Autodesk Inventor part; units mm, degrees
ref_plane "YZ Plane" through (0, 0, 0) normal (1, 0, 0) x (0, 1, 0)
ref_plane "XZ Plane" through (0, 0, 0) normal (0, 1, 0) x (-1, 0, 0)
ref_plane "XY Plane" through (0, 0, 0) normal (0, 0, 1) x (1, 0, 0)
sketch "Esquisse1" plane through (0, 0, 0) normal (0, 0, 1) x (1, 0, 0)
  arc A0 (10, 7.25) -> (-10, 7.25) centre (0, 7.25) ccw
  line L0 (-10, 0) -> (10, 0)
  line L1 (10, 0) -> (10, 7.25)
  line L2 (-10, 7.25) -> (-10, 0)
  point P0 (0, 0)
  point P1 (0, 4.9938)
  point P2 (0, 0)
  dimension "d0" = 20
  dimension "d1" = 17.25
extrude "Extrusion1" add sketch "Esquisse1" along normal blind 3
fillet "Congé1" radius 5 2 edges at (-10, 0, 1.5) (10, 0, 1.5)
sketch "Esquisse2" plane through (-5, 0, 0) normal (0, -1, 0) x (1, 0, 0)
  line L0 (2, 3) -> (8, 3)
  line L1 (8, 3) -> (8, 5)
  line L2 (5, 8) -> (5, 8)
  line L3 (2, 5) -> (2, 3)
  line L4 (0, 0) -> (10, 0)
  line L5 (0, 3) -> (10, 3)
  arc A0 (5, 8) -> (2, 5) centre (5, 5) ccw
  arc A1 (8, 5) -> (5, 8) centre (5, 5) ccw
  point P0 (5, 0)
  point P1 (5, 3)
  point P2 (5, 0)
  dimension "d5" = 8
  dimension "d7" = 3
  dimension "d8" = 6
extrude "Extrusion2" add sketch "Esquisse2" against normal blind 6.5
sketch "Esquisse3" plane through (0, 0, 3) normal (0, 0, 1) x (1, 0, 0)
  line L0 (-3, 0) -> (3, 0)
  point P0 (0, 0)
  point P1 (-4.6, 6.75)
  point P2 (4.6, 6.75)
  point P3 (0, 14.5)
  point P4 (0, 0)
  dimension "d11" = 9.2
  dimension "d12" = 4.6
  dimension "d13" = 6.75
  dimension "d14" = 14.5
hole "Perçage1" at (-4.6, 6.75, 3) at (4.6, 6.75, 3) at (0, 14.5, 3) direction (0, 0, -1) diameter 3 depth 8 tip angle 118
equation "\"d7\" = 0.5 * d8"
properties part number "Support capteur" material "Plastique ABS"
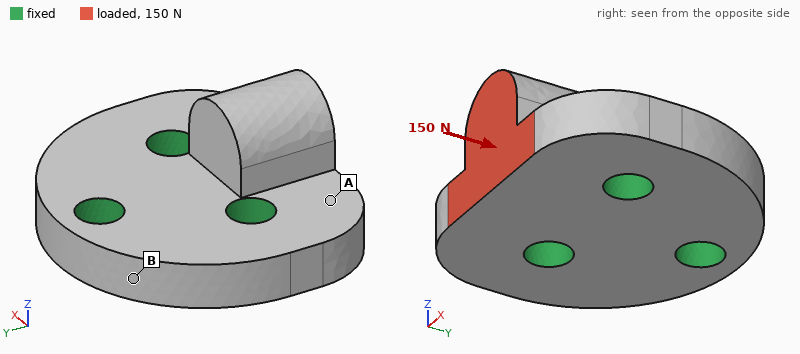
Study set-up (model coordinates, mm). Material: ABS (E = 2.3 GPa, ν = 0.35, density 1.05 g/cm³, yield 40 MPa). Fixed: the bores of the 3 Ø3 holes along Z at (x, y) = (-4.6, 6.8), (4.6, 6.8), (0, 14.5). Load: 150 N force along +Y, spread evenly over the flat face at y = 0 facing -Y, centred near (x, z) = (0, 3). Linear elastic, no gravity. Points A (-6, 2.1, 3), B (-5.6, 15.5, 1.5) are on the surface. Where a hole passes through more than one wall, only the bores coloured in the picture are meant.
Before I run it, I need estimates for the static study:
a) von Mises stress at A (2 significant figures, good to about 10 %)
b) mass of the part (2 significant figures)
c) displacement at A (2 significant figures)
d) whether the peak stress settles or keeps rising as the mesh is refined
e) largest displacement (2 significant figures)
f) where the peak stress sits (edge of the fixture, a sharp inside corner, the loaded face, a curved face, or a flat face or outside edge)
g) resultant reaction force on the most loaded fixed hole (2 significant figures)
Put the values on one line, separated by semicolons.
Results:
3.4 MPa; 1.0 g; 16 µm; keeps rising; 74 µm; edge of the fixture; 72 N
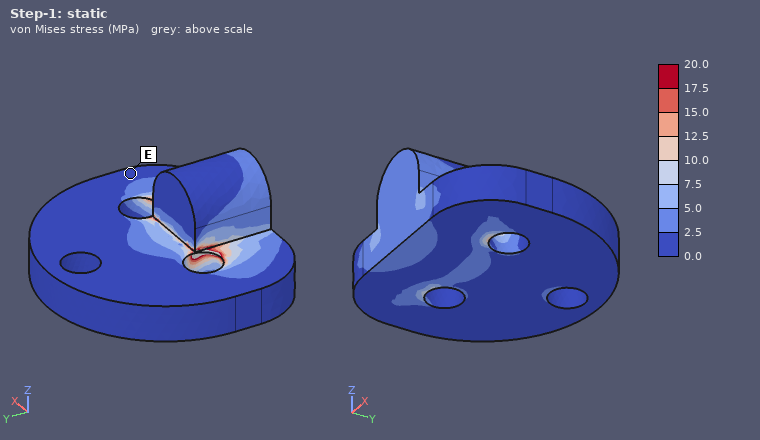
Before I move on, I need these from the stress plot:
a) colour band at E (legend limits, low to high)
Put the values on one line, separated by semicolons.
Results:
0.0 to 2.5 MPa
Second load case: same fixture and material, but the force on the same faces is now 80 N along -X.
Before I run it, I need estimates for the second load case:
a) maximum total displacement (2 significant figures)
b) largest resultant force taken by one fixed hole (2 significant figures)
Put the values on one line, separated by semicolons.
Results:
28 µm; 63 N
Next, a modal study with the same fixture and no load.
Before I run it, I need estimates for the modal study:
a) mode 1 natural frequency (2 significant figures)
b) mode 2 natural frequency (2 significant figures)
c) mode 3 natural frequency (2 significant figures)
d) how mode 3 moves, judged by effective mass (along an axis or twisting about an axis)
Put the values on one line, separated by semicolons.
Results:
11 kHz; 20 kHz; 22 kHz; twisting about Y
